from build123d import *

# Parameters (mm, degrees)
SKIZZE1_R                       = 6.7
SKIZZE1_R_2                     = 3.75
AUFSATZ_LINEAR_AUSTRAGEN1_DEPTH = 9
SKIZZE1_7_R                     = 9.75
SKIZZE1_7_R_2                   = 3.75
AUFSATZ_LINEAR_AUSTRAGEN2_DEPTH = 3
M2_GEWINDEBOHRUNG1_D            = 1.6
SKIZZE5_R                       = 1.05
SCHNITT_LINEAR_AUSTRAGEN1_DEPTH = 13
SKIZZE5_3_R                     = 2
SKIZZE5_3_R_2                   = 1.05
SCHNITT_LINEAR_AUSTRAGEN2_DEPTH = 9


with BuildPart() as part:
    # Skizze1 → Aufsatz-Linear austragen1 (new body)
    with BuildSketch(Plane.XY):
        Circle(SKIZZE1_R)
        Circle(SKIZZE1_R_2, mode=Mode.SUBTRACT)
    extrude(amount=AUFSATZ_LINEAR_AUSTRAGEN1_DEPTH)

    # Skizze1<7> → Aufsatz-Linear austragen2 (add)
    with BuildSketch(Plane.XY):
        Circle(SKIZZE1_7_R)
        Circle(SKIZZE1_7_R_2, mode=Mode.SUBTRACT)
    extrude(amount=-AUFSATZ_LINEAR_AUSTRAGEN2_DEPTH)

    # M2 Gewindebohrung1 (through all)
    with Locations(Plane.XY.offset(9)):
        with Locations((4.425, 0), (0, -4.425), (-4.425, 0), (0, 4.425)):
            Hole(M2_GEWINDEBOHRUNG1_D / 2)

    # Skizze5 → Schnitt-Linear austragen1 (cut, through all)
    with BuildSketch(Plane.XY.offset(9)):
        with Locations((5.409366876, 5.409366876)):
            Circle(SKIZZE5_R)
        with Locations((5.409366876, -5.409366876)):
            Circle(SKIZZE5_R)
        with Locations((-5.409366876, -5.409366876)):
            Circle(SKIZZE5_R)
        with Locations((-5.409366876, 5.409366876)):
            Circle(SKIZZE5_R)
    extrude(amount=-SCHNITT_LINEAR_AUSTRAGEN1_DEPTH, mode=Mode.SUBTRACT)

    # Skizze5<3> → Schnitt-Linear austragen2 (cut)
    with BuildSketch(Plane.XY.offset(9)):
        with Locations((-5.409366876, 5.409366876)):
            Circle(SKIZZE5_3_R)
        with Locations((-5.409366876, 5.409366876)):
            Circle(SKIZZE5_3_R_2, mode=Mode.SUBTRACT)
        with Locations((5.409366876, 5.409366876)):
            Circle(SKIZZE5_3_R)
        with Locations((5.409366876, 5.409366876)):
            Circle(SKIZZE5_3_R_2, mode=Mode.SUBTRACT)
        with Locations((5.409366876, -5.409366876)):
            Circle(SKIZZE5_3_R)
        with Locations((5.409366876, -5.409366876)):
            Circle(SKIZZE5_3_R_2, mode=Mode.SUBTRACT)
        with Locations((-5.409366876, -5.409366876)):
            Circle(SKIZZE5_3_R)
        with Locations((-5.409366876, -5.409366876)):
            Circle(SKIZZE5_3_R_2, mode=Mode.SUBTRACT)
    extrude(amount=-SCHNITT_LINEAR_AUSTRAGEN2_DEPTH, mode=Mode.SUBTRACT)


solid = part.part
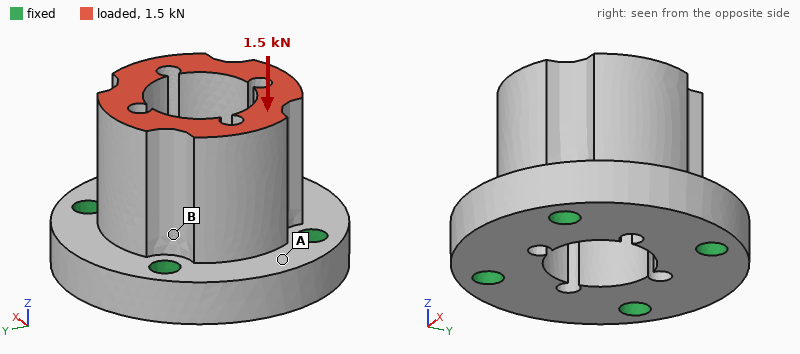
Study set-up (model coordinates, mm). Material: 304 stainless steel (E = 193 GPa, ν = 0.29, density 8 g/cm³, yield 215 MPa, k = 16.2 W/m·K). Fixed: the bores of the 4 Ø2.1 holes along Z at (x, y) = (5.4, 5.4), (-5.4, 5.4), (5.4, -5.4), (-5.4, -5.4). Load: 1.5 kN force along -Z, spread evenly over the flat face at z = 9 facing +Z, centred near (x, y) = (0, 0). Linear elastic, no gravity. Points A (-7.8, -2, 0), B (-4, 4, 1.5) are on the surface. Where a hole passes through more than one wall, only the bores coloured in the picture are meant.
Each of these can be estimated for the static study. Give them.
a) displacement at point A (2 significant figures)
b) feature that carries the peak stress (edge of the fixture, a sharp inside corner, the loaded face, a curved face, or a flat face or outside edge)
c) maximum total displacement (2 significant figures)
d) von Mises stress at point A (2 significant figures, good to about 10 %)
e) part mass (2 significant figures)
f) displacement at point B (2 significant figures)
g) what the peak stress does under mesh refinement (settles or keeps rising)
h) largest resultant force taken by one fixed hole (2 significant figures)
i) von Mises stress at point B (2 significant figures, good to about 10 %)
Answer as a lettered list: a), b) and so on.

a) 0.54 µm
b) edge of the fixture
c) 1.7 µm
d) 10 MPa
e) 11 g
f) 0.98 µm
g) keeps rising
h) 380 N
i) 27 MPa
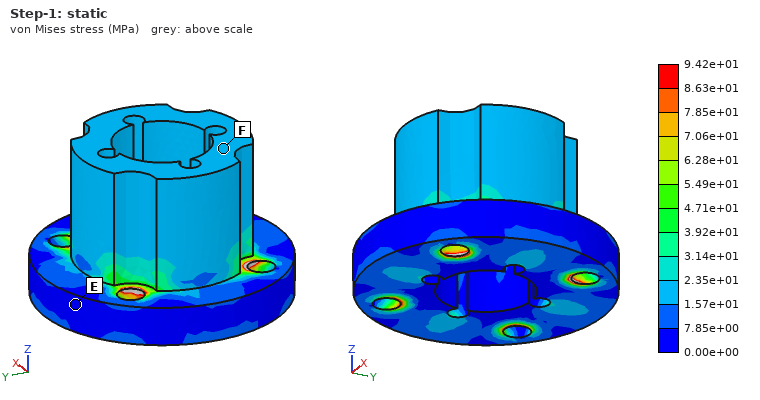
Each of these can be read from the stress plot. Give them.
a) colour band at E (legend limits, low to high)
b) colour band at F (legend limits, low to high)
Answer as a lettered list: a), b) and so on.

a) 0.00e+00 to 7.85e+00 MPa
b) 1.57e+01 to 2.35e+01 MPa
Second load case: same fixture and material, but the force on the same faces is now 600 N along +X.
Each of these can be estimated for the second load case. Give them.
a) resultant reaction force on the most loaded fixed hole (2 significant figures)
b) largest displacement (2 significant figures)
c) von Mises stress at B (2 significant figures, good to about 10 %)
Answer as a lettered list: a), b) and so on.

a) 320 N
b) 5.5 µm
c) 31 MPa
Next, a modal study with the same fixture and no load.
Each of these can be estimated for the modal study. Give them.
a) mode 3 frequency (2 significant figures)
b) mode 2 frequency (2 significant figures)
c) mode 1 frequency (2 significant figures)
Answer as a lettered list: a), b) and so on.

a) 41 kHz
b) 38 kHz
c) 38 kHz
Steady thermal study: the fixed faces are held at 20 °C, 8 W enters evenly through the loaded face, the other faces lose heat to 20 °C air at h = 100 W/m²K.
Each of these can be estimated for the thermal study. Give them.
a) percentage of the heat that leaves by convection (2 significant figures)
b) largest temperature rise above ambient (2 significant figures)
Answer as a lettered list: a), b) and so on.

a) 34 %
b) 57 K
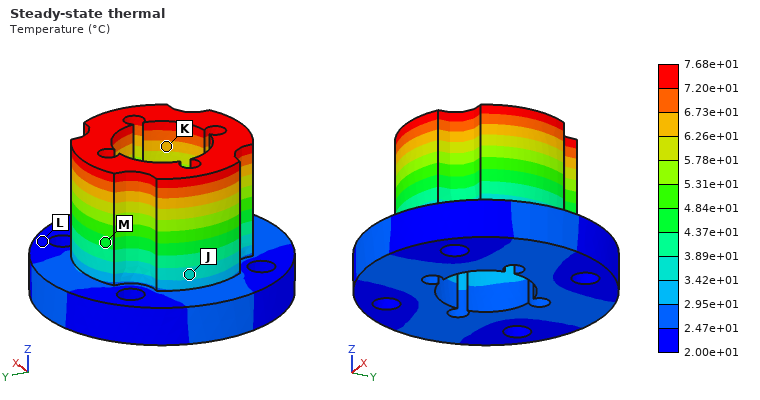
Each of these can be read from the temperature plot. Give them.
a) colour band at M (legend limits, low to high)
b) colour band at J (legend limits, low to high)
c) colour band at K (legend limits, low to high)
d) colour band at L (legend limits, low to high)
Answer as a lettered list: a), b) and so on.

a) 4.37e+01 to 4.84e+01 °C
b) 3.42e+01 to 3.89e+01 °C
c) 6.26e+01 to 6.73e+01 °C
d) 2.00e+01 to 2.47e+01 °C
